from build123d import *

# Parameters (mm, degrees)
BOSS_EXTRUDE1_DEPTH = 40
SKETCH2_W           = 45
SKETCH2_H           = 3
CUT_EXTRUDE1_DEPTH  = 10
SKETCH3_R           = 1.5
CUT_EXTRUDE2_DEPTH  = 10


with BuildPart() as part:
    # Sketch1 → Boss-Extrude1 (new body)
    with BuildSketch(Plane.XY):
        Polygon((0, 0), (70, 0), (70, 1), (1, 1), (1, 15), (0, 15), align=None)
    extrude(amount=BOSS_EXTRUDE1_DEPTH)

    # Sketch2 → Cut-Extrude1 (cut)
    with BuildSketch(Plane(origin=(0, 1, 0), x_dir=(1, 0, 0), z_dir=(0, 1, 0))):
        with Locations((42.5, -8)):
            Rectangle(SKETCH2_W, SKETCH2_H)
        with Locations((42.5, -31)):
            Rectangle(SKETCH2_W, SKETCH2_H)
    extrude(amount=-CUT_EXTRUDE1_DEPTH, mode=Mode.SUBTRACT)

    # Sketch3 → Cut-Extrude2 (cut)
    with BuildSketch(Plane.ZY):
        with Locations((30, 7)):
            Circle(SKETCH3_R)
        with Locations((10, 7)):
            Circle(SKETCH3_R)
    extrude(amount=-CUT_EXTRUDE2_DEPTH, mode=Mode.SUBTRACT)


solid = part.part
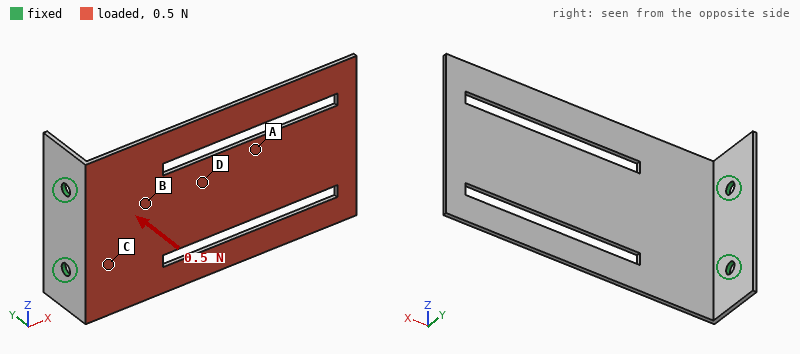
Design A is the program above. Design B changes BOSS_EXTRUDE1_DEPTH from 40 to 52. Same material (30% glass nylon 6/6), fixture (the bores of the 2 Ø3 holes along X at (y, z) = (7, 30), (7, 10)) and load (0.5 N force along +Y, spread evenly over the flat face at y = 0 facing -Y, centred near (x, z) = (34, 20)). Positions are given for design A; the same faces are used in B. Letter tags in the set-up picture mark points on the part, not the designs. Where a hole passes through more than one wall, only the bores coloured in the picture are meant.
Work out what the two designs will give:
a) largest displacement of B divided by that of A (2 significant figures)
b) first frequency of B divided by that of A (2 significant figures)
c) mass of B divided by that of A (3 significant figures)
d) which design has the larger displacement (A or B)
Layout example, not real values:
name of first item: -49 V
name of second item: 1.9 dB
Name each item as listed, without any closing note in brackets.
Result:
largest displacement of B divided by that of A: 0.83
first frequency of B divided by that of A: 0.96
mass of B divided by that of A: 1.33
which design has the larger displacement: A
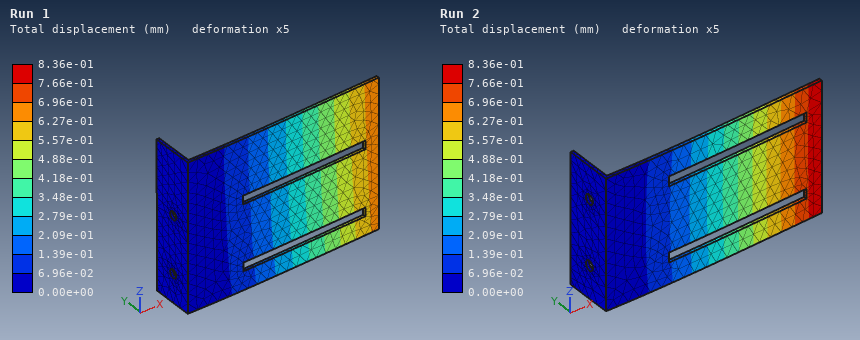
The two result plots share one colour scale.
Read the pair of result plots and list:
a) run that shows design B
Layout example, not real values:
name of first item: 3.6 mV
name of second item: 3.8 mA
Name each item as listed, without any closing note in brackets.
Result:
run that shows design B: Run 1
